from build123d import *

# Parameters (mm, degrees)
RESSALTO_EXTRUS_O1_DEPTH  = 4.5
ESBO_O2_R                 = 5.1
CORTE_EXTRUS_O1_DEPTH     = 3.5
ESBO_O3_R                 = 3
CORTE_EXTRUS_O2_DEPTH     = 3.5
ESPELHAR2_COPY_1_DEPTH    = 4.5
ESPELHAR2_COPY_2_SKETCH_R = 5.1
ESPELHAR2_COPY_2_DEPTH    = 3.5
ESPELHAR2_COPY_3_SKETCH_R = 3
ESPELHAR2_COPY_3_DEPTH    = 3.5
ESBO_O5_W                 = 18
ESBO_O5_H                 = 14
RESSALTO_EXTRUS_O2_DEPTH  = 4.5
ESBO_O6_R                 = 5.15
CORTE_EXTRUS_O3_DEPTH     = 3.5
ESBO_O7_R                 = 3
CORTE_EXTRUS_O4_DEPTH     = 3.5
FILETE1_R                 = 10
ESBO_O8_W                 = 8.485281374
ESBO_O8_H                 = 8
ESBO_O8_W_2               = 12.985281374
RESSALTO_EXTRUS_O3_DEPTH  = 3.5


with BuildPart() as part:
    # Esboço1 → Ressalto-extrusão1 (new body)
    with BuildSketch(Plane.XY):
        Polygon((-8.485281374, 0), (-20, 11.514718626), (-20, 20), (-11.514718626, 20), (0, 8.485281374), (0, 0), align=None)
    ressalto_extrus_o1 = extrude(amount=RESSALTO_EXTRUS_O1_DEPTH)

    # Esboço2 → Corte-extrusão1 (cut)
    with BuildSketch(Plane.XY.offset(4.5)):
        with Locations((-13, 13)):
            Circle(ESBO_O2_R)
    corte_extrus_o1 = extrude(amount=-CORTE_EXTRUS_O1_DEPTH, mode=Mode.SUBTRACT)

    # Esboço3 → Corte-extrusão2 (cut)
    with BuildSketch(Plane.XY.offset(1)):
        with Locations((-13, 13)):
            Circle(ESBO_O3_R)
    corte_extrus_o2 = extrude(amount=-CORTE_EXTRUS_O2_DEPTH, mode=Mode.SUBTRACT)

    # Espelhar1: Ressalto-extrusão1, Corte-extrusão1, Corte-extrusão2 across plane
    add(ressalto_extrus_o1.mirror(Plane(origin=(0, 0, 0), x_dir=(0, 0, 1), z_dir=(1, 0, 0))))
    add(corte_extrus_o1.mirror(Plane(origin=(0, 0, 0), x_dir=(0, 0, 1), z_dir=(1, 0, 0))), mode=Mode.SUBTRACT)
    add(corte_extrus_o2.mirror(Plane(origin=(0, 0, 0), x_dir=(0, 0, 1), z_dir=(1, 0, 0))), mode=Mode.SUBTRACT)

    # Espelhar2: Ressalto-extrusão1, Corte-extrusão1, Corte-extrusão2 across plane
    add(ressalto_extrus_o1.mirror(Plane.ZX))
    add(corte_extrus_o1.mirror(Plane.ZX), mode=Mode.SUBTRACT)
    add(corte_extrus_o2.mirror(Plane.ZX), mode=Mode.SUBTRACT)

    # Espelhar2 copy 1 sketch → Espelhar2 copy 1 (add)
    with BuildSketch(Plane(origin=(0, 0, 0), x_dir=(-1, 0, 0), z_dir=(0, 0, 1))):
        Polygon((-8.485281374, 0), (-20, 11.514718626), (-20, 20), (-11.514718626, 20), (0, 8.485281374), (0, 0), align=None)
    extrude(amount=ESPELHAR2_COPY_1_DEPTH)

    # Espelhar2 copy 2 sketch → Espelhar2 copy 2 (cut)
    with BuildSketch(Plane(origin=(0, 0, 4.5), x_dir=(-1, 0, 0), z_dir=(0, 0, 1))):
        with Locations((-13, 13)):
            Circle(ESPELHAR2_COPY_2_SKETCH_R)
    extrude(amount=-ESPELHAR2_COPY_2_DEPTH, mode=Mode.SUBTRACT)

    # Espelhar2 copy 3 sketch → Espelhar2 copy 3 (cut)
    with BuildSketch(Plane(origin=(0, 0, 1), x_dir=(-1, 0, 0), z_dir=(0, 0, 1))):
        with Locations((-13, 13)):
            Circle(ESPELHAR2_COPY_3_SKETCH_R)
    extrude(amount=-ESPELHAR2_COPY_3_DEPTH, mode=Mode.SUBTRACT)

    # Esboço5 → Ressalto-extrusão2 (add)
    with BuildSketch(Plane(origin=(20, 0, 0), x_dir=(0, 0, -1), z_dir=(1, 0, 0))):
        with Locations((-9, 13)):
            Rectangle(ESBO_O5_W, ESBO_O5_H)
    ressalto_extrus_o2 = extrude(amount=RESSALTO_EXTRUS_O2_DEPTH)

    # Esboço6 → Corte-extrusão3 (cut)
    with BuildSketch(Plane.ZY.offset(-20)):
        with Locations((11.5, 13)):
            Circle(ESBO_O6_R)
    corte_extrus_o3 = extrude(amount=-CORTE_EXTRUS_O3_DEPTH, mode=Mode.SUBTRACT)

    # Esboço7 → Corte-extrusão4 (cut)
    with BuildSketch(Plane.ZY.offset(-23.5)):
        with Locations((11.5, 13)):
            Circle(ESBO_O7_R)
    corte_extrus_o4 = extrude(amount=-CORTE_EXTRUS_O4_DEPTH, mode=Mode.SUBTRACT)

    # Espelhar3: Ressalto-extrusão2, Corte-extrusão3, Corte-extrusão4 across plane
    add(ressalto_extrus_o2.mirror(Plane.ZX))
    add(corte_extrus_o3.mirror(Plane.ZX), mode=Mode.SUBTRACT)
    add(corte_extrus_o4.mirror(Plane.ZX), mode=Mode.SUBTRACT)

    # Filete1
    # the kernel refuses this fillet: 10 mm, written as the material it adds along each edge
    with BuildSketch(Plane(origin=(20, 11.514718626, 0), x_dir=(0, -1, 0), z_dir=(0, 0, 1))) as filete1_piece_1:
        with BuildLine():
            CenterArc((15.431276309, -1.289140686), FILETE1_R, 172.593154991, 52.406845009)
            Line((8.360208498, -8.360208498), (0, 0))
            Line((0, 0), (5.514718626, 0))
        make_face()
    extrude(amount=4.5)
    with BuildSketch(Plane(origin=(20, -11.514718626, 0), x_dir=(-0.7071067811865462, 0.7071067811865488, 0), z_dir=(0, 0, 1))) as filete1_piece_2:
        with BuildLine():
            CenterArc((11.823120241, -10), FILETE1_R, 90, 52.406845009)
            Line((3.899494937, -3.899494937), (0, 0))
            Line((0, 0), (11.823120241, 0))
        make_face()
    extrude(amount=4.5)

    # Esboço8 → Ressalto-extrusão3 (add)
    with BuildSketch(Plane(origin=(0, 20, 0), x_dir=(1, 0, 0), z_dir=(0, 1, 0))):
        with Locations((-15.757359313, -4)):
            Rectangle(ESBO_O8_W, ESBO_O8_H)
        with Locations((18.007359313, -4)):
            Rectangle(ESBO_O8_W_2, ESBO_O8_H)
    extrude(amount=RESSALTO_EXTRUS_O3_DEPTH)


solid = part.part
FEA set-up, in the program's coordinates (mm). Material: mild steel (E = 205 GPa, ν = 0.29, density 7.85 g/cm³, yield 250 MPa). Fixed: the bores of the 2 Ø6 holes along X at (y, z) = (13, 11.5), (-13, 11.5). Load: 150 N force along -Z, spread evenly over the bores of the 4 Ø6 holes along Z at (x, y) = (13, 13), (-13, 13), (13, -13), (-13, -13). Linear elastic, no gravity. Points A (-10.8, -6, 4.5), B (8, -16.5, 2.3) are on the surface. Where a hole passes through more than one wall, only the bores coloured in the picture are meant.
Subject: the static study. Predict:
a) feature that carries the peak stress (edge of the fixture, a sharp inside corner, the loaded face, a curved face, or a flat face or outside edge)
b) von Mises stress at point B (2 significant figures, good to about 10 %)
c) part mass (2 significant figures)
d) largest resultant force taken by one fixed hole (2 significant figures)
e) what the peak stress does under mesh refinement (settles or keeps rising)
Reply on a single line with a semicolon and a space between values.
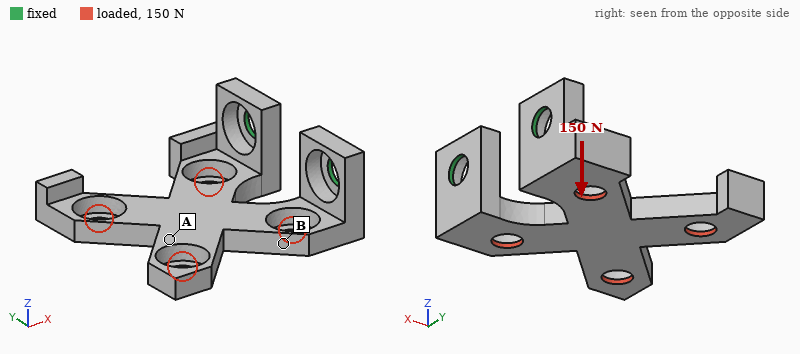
edge of the fixture; 47 MPa; 47 g; 79 N; keeps rising
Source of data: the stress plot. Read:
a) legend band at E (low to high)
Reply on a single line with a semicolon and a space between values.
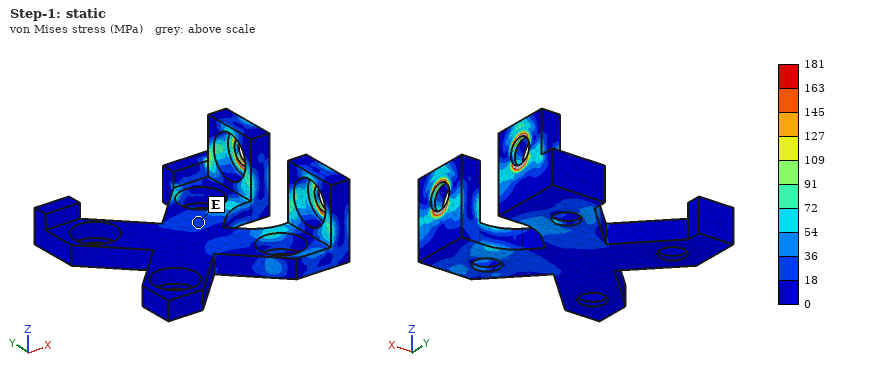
18 to 36 MPa
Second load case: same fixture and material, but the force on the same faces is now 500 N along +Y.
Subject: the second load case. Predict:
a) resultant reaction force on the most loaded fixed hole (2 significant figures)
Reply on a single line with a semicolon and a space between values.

470 N
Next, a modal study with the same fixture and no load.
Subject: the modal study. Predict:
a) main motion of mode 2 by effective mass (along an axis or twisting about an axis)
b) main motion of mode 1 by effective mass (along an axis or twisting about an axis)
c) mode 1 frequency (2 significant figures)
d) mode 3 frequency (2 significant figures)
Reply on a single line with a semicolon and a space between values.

along Y; along Z; 1100 Hz; 3900 Hz
